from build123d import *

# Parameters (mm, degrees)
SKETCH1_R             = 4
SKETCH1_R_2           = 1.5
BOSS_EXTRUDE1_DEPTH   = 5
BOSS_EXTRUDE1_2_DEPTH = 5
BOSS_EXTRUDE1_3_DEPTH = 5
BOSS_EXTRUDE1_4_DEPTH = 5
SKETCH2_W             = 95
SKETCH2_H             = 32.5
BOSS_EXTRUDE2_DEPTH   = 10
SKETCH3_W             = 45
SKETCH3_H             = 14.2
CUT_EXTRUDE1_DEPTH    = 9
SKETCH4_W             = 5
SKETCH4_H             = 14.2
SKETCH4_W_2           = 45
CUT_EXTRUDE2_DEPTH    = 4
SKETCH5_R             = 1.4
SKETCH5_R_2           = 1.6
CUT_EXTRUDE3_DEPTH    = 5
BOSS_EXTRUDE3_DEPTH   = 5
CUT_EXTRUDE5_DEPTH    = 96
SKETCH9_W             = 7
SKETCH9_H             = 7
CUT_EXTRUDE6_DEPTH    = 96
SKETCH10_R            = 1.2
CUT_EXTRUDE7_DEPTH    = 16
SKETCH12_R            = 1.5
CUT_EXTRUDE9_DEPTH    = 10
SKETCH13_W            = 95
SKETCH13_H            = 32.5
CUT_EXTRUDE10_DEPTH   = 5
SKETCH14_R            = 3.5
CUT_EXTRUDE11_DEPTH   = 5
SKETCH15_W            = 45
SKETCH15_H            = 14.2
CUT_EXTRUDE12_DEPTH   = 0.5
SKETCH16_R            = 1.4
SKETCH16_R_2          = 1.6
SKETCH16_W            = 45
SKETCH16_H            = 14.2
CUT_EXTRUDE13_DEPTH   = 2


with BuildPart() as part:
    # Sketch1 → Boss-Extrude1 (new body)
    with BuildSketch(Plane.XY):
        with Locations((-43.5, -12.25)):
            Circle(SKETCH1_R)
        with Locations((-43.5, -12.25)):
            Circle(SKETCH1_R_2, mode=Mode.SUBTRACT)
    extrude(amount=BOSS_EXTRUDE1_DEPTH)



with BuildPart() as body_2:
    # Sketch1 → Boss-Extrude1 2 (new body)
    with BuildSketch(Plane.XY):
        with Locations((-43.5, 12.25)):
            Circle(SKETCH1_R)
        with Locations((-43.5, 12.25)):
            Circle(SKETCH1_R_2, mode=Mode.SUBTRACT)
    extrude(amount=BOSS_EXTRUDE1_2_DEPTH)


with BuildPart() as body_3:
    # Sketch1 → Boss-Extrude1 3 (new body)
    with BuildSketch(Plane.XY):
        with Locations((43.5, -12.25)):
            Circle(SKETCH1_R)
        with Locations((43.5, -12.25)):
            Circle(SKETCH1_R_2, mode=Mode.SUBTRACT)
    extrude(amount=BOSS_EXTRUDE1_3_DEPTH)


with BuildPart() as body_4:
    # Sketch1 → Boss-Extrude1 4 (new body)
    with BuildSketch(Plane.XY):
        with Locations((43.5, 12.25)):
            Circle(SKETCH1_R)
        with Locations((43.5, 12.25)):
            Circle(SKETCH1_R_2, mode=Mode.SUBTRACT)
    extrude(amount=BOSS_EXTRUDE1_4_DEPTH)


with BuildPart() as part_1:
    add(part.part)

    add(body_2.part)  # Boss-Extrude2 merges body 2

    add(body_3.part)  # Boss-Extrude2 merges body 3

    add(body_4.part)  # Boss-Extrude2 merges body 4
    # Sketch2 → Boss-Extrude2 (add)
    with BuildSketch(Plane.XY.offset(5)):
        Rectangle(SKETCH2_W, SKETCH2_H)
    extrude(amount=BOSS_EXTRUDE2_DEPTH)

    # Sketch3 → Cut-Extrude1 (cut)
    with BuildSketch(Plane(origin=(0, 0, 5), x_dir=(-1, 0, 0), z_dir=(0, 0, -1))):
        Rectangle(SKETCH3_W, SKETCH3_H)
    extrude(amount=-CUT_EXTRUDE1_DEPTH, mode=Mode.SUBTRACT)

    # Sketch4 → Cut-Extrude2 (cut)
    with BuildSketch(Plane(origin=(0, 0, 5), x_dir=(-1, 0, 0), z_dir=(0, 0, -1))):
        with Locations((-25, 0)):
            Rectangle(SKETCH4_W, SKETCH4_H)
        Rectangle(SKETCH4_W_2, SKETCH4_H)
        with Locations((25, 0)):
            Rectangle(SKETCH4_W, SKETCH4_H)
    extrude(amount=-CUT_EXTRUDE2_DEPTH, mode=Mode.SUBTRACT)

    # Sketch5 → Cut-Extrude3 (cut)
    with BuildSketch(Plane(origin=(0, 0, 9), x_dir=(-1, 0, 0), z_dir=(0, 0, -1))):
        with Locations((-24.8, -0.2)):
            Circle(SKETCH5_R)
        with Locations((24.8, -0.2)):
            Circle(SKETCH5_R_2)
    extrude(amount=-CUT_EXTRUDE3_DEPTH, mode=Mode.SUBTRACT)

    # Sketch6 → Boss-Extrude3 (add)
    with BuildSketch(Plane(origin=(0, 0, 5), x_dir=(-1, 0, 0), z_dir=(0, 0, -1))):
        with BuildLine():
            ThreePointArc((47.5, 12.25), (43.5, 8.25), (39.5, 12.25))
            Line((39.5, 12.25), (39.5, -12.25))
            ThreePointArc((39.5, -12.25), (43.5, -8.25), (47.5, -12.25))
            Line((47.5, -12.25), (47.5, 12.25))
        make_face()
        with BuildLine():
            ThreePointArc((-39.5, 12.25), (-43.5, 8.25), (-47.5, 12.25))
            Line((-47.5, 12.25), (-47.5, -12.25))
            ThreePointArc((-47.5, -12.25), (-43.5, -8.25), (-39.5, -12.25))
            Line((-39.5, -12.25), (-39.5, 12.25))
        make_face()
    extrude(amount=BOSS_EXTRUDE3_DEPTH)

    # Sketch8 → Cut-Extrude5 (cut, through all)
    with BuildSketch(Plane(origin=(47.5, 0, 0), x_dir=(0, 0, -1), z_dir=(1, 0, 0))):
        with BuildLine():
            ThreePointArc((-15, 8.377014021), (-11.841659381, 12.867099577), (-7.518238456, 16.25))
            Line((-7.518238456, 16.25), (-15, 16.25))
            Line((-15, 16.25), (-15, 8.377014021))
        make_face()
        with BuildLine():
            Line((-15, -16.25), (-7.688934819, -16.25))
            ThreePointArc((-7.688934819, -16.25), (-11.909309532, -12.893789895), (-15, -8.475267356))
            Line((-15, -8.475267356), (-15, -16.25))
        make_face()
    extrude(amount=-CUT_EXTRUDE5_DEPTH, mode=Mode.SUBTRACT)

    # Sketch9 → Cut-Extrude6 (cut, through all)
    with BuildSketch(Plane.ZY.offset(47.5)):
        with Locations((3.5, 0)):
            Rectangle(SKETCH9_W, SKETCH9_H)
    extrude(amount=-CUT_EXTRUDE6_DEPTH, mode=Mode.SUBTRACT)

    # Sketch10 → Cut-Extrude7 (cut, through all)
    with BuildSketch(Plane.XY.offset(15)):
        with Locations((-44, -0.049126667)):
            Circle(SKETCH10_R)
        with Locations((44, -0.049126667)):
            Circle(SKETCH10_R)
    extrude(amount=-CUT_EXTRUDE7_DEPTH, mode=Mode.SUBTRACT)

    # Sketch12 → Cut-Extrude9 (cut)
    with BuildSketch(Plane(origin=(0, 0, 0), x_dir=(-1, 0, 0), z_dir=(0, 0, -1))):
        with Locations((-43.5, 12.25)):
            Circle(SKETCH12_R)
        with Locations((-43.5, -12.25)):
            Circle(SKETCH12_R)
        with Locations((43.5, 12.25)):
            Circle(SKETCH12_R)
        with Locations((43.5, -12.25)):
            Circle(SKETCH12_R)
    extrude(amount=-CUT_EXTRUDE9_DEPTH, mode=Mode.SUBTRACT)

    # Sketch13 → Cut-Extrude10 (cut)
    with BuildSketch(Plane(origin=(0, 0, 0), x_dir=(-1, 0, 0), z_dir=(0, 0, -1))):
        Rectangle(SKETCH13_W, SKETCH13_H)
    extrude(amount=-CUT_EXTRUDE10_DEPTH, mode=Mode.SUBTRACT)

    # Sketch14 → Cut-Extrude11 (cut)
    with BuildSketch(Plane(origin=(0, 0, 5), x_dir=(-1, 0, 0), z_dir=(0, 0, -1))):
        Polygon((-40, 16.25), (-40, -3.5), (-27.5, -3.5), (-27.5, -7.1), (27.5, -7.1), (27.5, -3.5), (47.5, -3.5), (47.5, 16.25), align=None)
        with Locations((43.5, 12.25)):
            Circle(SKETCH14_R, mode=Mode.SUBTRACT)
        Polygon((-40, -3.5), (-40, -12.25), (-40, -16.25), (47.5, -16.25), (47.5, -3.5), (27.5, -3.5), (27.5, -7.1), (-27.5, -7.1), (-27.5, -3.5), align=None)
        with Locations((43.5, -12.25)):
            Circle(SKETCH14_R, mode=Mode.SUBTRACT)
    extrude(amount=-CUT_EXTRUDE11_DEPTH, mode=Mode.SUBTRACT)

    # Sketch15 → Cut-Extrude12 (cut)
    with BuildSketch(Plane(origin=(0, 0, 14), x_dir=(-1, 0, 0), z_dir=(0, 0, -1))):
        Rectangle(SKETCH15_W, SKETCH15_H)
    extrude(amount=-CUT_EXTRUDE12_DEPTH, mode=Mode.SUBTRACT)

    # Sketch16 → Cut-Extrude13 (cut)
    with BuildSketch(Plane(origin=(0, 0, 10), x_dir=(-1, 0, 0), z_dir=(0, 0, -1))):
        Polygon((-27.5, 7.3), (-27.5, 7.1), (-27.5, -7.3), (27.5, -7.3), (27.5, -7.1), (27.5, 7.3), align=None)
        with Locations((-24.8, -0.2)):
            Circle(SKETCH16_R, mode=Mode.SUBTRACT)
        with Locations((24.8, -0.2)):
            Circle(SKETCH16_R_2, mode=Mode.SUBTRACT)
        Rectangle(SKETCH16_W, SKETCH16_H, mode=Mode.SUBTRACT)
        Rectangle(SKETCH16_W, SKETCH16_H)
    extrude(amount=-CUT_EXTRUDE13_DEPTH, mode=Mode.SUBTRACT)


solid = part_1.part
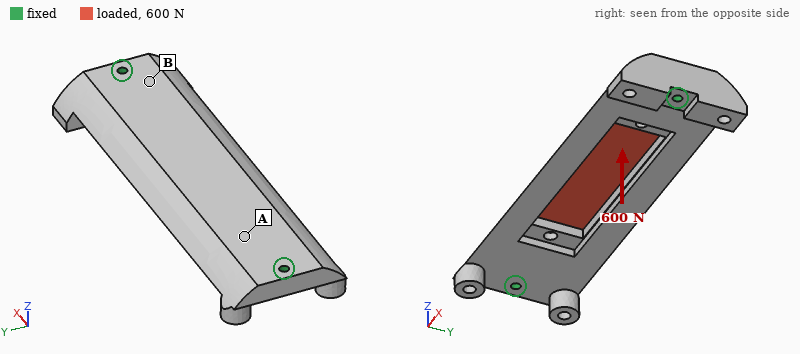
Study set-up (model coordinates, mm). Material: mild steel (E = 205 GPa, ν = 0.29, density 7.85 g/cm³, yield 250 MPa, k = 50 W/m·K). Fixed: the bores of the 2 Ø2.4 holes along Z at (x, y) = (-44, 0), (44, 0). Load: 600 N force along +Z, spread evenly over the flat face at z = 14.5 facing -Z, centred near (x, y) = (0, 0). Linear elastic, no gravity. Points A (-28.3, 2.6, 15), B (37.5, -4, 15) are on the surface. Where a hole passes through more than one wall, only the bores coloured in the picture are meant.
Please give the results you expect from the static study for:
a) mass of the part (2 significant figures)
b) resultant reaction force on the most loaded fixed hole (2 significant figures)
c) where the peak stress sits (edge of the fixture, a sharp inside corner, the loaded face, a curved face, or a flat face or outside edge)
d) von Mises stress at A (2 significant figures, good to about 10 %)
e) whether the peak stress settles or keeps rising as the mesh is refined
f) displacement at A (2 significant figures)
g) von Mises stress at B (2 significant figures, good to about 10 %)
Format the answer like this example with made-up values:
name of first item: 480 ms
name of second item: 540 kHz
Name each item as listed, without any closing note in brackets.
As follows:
mass of the part: 74 g
resultant reaction force on the most loaded fixed hole: 320 N
where the peak stress sits: edge of the fixture
von Mises stress at A: 18 MPa
whether the peak stress settles or keeps rising as the mesh is refined: keeps rising
displacement at A: 19 µm
von Mises stress at B: 52 MPa
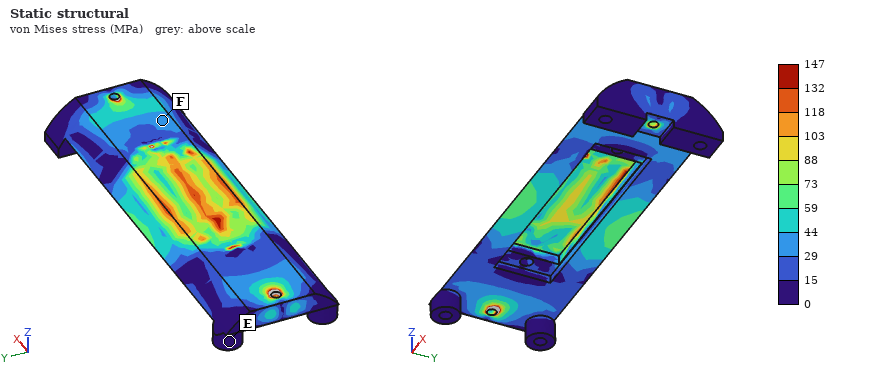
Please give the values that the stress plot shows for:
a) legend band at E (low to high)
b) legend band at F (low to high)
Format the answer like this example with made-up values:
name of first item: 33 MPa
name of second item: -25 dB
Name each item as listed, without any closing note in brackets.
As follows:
legend band at E: 0 to 15 MPa
legend band at F: 29 to 44 MPa
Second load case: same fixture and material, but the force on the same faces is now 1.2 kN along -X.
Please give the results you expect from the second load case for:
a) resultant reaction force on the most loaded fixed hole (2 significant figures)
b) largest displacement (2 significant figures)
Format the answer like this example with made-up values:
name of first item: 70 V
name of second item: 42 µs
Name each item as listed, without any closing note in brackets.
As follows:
resultant reaction force on the most loaded fixed hole: 610 N
largest displacement: 3.0 µm
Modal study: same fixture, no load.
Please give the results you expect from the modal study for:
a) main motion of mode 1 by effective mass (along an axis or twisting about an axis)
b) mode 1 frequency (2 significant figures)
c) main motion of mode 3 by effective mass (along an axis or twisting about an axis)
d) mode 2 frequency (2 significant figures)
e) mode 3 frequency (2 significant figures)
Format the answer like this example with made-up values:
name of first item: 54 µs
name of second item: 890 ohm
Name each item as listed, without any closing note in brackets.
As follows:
main motion of mode 1 by effective mass: along Z
mode 1 frequency: 3700 Hz
main motion of mode 3 by effective mass: along Y
mode 2 frequency: 4700 Hz
mode 3 frequency: 8400 Hz
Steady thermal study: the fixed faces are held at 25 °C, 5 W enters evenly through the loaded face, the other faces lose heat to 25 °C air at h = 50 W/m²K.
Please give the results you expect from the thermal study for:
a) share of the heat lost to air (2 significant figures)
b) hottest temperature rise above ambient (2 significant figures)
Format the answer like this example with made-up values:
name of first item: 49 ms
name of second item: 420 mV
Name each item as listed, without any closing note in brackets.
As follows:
share of the heat lost to air: 44 %
hottest temperature rise above ambient: 21 K
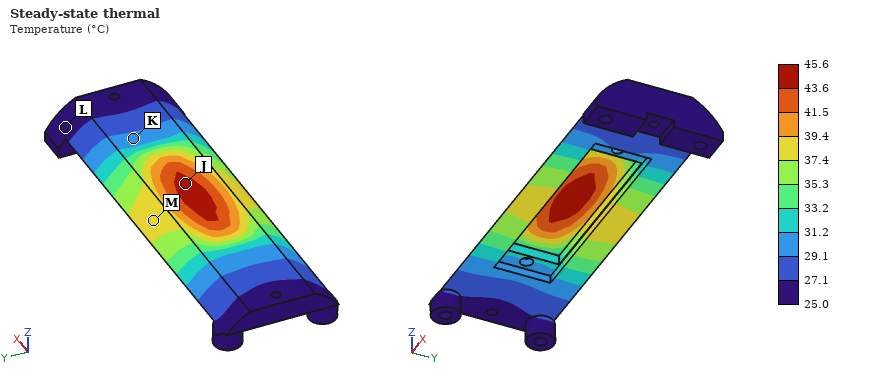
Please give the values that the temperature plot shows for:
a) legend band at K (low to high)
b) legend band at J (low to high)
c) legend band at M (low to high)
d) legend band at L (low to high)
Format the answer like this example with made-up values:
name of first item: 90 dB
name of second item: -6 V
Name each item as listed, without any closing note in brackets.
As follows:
legend band at K: 29.1 to 31.2 °C
legend band at J: 43.6 to 45.6 °C
legend band at M: 37.4 to 39.4 °C
legend band at L: 25.0 to 27.1 °C
